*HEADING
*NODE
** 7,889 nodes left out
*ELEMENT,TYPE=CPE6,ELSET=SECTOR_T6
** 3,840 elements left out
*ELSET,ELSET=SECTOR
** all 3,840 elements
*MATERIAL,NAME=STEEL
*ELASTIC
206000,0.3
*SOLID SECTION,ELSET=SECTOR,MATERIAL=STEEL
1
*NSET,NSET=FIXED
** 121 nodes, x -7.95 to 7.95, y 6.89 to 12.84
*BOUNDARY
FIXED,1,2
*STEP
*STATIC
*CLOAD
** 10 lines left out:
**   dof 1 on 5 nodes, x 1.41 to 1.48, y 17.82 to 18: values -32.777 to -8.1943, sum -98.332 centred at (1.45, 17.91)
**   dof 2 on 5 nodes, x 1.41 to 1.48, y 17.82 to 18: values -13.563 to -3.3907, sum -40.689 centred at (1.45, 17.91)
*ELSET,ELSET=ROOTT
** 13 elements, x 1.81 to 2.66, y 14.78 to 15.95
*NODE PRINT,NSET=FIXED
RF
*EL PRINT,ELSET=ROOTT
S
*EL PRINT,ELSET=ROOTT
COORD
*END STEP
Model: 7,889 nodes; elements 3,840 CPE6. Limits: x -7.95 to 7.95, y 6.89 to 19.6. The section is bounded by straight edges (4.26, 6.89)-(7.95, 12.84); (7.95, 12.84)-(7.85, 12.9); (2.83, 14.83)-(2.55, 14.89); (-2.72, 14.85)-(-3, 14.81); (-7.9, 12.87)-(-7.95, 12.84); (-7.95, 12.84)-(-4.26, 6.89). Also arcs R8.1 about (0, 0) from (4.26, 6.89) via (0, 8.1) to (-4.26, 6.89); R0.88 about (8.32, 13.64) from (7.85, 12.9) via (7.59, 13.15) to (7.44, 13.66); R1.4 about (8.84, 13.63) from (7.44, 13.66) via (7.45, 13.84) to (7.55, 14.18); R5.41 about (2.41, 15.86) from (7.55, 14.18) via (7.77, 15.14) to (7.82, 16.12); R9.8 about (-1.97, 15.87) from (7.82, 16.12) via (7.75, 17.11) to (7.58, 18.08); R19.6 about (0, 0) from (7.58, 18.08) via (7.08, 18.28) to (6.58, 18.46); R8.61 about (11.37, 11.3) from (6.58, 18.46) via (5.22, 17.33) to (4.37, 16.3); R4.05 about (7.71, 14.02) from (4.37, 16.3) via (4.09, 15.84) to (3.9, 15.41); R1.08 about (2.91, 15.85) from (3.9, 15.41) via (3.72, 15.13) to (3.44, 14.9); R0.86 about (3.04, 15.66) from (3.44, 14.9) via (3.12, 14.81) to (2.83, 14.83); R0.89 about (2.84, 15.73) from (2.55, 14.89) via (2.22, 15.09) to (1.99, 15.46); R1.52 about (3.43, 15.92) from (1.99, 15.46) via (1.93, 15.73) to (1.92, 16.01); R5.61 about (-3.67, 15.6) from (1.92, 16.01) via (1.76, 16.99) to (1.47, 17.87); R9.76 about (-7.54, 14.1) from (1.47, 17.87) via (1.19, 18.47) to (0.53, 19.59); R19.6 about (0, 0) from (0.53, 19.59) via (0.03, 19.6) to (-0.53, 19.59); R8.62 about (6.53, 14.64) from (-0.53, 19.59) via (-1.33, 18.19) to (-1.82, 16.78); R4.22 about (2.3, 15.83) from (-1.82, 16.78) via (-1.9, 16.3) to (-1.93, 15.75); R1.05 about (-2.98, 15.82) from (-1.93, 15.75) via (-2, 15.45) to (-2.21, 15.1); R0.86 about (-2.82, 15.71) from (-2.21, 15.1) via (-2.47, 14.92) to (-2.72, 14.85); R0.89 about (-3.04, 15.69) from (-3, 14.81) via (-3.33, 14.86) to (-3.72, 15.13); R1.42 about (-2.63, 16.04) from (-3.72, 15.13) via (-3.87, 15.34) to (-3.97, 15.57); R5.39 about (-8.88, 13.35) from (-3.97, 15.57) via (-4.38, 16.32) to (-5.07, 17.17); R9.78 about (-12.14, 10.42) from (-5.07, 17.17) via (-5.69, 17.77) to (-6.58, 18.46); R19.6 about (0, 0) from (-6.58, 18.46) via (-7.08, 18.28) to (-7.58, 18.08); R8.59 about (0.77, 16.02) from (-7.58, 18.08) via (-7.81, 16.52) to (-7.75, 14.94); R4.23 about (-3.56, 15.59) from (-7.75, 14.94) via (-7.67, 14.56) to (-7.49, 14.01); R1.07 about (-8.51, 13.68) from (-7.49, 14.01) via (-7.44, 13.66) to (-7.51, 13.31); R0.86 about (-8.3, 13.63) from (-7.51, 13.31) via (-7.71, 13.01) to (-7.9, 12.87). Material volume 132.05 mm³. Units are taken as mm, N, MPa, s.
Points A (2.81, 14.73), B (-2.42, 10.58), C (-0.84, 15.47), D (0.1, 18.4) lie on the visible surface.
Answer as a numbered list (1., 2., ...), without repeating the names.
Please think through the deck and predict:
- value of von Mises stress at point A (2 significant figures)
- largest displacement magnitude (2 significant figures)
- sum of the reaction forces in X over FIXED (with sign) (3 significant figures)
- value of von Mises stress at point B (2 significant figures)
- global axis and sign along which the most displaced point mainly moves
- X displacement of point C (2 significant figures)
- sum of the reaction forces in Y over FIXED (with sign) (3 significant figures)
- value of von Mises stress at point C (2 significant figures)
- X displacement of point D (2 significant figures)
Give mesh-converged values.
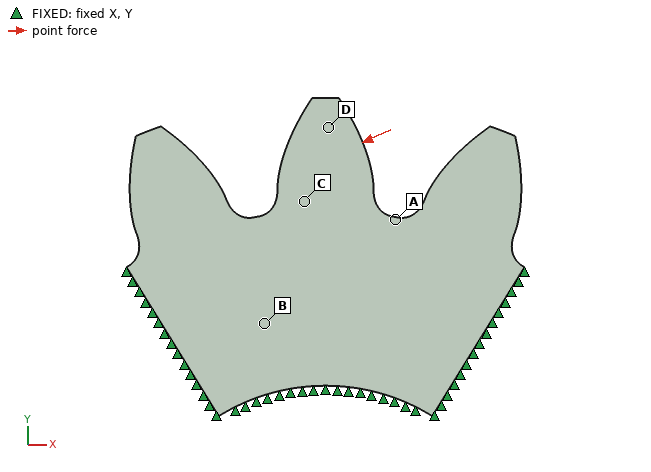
1. 46 MPa
2. 0.0037 mm
3. 98.3 N
4. 12 MPa
5. -X
6. -8.9e-04 mm
7. 40.7 N
8. 45 MPa
9. -0.0030 mm
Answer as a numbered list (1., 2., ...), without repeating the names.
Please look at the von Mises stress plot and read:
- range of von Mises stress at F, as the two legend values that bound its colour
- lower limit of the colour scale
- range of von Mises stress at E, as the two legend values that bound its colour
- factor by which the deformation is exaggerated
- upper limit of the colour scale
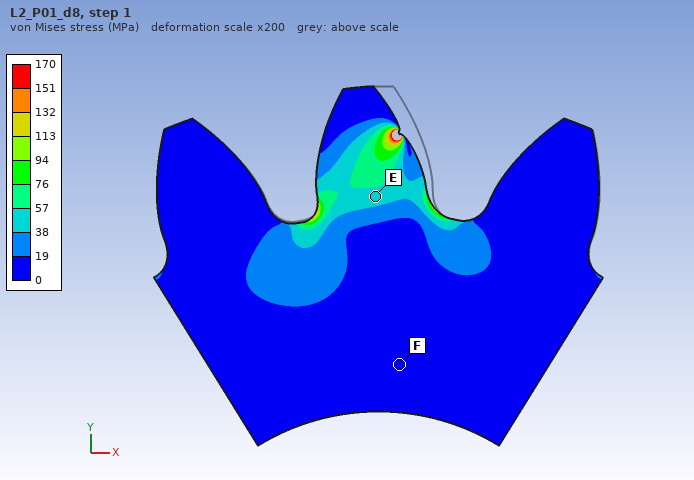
1. 0 to 19 MPa
2. 0 MPa
3. 38 to 57 MPa
4. 200
5. 170 MPa
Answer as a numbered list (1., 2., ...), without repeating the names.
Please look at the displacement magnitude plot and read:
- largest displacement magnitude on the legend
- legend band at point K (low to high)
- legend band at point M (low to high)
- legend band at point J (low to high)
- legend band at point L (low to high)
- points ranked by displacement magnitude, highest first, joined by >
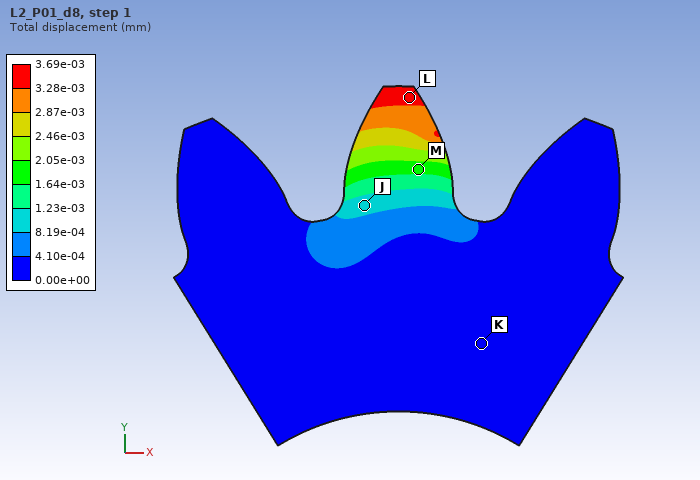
1. 3.69e-03 mm
2. 0.00e+00 to 4.10e-04 mm
3. 1.64e-03 to 2.05e-03 mm
4. 8.19e-04 to 1.23e-03 mm
5. 3.28e-03 to 3.69e-03 mm
6. L > M > J > K
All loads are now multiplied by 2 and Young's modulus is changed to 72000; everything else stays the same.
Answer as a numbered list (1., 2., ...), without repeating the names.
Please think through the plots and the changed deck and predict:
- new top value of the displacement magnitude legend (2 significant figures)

1. 0.021 mm
